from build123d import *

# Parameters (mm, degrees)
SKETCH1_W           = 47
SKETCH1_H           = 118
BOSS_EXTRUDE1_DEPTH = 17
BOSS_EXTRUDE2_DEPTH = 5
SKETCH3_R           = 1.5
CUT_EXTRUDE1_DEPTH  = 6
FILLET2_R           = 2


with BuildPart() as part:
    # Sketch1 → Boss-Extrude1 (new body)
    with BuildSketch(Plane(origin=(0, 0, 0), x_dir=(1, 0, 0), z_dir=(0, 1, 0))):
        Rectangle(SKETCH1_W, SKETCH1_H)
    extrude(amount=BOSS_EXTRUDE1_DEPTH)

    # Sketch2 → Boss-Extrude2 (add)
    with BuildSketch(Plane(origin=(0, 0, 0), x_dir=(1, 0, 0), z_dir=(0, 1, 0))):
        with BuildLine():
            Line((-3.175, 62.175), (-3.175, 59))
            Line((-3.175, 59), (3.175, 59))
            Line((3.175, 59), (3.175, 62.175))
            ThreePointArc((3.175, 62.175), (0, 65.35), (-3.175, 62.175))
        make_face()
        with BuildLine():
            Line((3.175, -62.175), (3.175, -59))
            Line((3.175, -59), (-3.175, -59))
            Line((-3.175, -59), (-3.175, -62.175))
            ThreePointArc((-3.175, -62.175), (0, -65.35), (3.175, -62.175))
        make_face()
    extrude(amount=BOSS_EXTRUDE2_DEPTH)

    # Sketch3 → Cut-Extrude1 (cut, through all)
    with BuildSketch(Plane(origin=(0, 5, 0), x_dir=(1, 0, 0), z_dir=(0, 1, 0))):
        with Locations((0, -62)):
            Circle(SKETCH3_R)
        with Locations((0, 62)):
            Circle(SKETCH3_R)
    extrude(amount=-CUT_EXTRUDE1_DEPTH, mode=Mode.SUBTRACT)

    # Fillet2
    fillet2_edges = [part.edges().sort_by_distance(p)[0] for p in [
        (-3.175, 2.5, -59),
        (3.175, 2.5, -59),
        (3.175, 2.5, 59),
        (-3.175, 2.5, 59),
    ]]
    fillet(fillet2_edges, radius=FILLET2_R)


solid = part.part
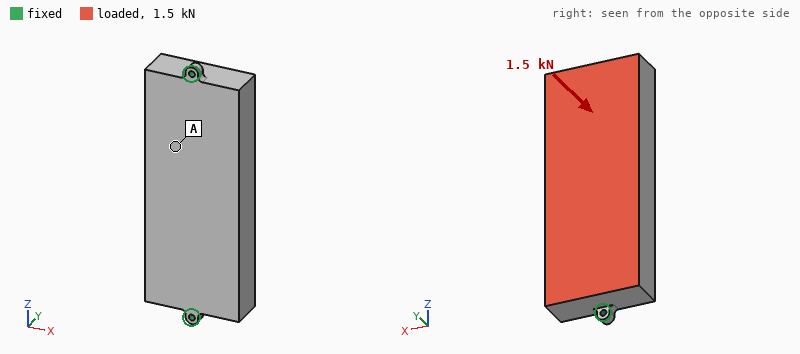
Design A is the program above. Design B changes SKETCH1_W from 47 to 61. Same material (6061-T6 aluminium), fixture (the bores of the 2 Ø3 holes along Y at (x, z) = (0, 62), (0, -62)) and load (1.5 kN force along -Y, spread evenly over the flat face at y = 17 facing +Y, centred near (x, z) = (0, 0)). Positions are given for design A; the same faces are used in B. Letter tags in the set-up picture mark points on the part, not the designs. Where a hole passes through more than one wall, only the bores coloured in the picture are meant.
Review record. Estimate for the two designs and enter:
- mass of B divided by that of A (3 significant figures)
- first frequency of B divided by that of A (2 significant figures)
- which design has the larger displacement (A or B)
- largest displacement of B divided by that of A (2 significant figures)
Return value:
1.30
0.71
A
0.89
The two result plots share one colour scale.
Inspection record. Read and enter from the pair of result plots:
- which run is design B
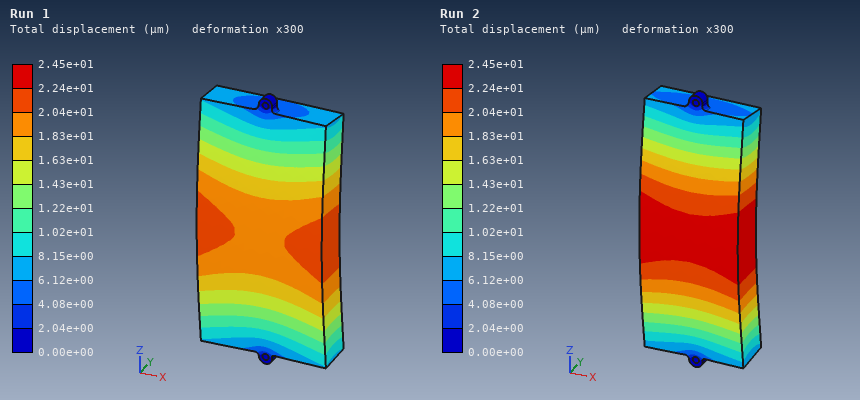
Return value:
Run 1
